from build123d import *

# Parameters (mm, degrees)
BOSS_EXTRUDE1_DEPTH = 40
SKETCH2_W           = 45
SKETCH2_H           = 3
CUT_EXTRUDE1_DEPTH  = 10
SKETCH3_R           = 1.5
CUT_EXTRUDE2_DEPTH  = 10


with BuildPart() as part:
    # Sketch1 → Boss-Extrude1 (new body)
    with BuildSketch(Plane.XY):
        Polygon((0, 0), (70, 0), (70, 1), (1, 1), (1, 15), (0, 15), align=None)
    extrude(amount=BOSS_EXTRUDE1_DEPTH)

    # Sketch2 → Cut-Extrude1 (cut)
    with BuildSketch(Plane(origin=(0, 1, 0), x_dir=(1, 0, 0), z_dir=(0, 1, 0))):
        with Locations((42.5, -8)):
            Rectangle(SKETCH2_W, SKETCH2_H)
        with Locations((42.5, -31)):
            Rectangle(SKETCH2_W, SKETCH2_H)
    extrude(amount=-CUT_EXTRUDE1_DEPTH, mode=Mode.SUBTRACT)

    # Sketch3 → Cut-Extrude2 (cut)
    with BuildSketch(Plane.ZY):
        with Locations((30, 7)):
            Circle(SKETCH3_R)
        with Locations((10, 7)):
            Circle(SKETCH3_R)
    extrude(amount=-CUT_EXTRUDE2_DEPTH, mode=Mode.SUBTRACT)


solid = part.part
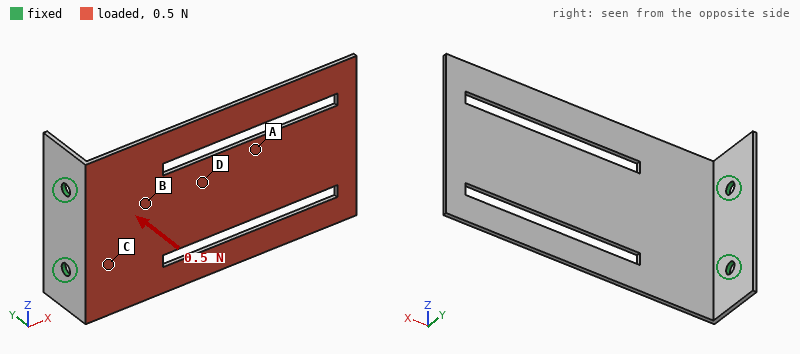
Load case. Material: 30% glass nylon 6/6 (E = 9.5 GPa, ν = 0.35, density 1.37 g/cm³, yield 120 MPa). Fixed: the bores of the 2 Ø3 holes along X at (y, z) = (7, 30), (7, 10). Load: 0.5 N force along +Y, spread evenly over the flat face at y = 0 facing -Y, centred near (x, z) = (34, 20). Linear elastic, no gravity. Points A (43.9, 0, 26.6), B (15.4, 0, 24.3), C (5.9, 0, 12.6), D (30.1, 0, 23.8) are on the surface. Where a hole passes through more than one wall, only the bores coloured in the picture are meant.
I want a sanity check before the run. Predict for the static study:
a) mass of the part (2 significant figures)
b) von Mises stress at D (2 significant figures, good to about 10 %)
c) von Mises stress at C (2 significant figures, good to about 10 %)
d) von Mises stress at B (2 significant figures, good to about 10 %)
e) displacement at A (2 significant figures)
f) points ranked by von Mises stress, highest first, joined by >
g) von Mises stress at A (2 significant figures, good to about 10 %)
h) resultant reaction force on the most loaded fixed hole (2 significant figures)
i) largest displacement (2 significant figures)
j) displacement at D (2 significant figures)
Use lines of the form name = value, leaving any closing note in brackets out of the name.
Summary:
mass of the part = 4.2 g
von Mises stress at D = 0.94 MPa
von Mises stress at C = 2.0 MPa
von Mises stress at B = 1.4 MPa
displacement at A = 0.44 mm
points ranked by von Mises stress, highest first, joined by > = C > B > D > A
von Mises stress at A = 0.43 MPa
resultant reaction force on the most loaded fixed hole = 0.26 N
largest displacement = 0.84 mm
displacement at D = 0.25 mm
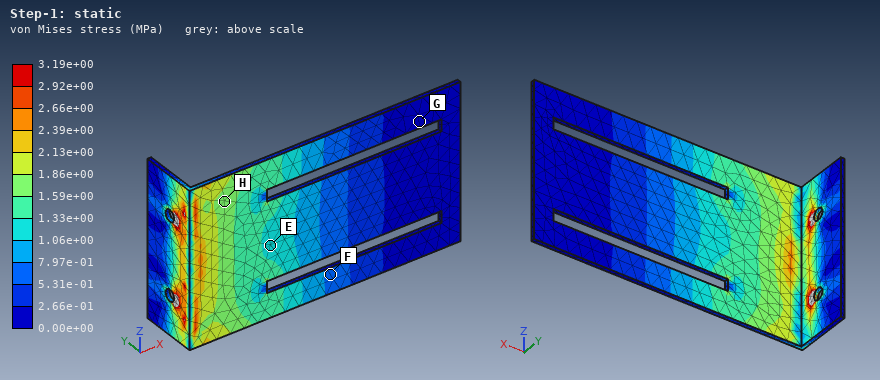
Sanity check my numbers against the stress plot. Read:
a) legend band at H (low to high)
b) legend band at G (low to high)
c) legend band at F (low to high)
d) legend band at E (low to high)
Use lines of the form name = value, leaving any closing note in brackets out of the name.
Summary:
legend band at H = 1.59e+00 to 1.86e+00 MPa
legend band at G = 0.00e+00 to 2.66e-01 MPa
legend band at F = 5.31e-01 to 7.97e-01 MPa
legend band at E = 1.06e+00 to 1.33e+00 MPa
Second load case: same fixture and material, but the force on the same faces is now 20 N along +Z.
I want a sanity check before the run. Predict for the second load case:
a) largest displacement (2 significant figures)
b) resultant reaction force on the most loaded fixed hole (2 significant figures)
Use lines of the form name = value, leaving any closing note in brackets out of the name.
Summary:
largest displacement = 0.87 mm
resultant reaction force on the most loaded fixed hole = 32 N
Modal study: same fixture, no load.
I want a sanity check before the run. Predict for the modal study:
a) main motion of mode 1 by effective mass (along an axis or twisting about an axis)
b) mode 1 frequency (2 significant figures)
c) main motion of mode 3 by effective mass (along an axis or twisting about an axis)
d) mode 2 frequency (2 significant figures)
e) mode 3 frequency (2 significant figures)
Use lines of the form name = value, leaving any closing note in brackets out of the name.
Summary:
main motion of mode 1 by effective mass = along Y
mode 1 frequency = 82 Hz
main motion of mode 3 by effective mass = along Y
mode 2 frequency = 310 Hz
mode 3 frequency = 490 Hz
